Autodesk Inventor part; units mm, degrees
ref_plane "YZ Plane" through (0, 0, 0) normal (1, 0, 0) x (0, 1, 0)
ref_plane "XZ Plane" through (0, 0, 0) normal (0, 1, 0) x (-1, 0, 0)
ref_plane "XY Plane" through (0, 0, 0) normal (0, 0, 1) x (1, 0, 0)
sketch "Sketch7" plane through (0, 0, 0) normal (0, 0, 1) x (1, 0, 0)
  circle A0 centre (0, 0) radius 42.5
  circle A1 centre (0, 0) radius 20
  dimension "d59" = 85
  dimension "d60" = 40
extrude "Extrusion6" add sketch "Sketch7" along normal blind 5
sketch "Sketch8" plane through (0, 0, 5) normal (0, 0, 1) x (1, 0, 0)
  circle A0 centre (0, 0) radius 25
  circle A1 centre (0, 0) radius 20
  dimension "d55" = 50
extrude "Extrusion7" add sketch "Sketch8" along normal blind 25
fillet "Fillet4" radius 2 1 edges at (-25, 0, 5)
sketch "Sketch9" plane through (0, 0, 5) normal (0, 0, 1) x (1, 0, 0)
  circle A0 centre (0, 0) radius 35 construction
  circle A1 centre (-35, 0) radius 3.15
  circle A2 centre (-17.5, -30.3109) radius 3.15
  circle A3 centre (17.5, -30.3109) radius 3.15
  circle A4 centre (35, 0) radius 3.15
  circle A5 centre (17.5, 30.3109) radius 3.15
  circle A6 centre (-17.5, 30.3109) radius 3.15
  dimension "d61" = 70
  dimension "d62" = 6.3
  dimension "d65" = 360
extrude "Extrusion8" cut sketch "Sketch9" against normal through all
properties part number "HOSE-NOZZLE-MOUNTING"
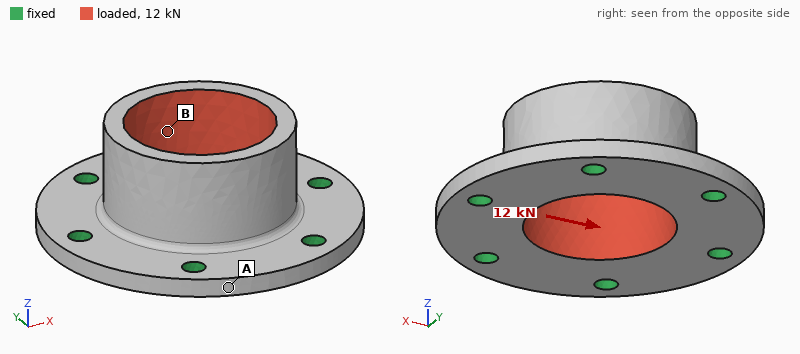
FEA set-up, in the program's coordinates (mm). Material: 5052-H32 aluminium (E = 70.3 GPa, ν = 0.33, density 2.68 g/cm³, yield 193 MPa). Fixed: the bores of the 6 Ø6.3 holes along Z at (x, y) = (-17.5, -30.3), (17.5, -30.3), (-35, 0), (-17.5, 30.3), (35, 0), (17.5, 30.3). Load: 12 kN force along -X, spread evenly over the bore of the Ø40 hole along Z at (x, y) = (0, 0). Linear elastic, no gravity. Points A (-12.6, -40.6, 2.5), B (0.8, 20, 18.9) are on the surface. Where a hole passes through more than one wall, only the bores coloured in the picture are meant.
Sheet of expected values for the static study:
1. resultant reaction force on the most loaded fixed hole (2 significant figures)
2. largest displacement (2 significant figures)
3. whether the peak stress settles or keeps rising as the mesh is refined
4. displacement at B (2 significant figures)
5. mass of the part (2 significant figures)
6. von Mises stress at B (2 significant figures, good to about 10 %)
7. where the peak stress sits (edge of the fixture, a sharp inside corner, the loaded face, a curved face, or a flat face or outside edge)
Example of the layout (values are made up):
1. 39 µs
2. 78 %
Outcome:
1. 3.0 kN
2. 42 µm
3. keeps rising
4. 23 µm
5. 100 g
6. 30 MPa
7. edge of the fixture
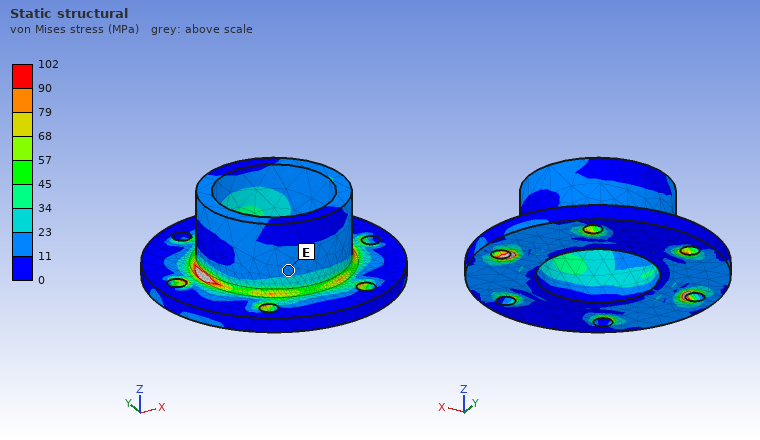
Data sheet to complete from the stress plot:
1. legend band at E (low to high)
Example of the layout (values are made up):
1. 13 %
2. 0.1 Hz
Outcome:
1. 11 to 23 MPa
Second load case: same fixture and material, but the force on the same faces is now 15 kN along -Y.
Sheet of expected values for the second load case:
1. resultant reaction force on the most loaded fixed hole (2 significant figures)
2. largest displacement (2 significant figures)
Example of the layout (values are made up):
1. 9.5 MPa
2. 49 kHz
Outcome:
1. 3.4 kN
2. 53 µm
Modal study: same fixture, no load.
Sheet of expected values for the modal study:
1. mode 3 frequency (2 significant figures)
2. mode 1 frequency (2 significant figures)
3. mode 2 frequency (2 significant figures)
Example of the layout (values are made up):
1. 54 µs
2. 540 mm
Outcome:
1. 12 kHz
2. 12 kHz
3. 12 kHz
